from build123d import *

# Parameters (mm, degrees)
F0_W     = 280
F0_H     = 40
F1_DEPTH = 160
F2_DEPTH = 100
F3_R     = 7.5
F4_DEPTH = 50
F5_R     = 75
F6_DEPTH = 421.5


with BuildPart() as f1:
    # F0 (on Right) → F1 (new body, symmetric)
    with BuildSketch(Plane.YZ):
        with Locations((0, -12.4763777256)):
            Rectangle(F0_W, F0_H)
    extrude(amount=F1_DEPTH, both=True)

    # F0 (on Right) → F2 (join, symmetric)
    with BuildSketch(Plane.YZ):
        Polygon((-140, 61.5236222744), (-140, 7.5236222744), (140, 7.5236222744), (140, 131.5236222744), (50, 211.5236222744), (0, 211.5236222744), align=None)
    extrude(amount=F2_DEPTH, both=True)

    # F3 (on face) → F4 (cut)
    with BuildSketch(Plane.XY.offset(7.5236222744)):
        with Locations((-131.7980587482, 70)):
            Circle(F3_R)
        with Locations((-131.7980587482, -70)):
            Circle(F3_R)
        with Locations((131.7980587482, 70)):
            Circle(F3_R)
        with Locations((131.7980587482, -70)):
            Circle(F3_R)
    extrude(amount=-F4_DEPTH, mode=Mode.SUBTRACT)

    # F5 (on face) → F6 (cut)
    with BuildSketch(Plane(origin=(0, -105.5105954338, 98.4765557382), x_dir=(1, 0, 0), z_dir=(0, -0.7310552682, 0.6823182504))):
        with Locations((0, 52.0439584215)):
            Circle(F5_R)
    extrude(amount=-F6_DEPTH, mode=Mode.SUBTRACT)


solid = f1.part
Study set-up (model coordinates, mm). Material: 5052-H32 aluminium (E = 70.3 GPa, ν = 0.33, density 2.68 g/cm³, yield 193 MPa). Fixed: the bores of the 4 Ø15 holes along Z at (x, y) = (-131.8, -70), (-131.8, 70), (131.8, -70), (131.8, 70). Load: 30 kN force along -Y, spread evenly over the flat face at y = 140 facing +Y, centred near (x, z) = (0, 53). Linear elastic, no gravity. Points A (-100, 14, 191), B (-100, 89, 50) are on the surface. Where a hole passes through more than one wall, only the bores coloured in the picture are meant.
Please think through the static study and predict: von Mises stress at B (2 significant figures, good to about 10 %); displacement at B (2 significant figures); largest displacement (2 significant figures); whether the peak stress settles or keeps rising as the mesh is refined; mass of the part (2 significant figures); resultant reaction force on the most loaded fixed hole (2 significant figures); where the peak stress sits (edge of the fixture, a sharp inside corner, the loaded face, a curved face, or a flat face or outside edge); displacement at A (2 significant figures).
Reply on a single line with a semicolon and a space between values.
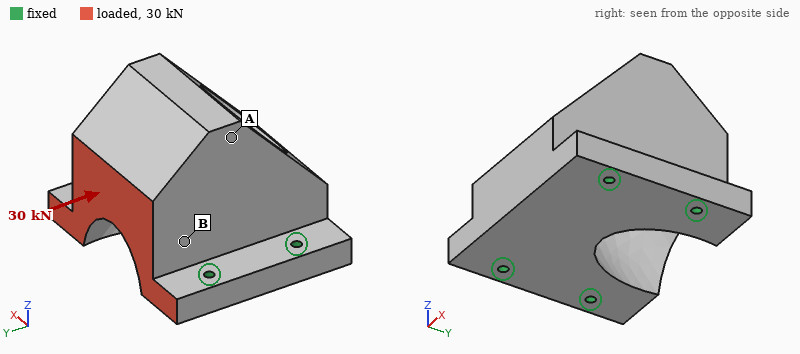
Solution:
3.7 MPa; 17 µm; 35 µm; keeps rising; 22 kg; 11 kN; edge of the fixture; 31 µm
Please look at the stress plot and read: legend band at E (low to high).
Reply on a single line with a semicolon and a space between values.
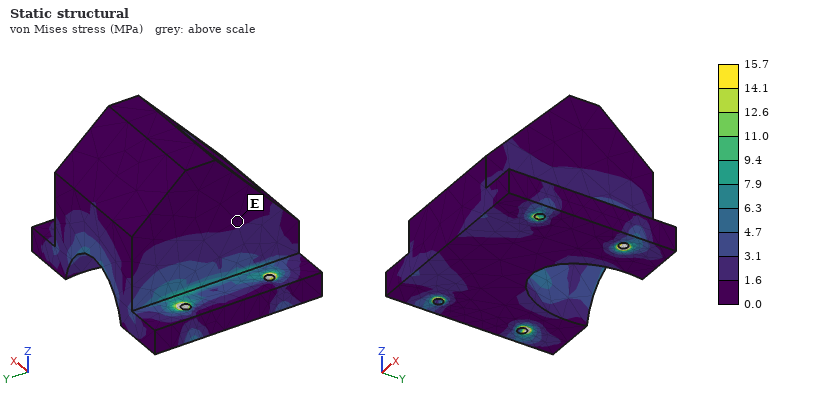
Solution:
0.0 to 1.6 MPa
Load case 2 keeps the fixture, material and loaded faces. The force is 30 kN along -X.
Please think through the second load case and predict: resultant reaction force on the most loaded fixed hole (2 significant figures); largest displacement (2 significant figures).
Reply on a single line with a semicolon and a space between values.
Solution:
17 kN; 35 µm
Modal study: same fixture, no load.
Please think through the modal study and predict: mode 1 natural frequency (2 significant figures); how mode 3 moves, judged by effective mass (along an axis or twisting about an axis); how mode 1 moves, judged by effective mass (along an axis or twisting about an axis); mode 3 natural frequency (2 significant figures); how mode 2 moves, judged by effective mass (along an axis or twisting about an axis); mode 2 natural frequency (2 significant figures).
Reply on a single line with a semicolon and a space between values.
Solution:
1100 Hz; along Z; along Y; 2000 Hz; along X; 1400 Hz
